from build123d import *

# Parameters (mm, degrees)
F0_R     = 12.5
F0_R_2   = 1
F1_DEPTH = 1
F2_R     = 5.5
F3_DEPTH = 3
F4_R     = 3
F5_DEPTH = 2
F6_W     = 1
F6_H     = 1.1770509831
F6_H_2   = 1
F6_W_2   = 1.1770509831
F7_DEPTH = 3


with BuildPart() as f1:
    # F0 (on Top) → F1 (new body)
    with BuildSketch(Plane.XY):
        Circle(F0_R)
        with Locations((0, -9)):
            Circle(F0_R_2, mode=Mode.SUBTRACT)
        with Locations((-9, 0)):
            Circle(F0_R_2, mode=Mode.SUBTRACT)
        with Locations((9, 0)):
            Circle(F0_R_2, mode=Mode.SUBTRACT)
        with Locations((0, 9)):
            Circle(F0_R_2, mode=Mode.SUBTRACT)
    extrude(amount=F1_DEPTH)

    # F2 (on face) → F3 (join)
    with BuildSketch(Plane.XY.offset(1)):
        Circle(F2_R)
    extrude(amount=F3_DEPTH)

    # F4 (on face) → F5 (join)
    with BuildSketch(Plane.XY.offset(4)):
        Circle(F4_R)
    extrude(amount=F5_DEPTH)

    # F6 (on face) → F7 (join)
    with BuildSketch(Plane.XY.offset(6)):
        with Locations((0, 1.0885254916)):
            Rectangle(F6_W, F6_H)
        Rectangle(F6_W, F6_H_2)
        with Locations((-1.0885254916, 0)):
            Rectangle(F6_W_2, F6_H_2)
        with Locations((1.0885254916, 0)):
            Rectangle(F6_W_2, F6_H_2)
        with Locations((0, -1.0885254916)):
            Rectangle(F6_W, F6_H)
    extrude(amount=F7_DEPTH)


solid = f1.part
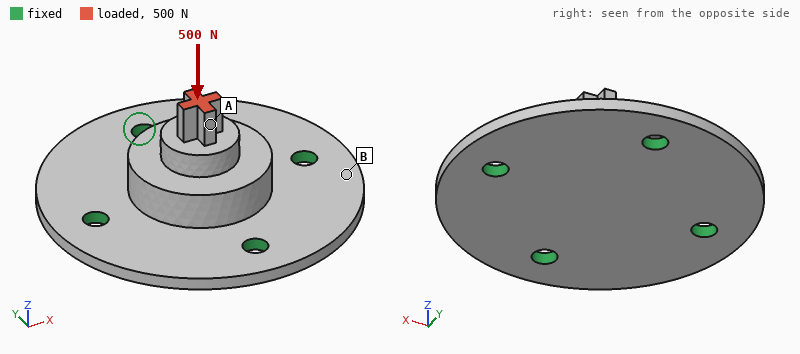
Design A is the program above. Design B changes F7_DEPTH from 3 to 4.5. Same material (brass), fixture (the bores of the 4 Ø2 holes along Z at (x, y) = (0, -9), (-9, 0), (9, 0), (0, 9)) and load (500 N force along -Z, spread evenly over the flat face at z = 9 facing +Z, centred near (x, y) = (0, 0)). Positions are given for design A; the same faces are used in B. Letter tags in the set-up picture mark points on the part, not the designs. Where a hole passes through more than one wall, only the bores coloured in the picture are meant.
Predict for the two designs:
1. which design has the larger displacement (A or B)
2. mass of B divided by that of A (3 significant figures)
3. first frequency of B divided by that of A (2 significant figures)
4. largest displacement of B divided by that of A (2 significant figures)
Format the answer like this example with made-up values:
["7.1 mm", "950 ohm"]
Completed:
["B", "1.01", "1.00", "1.1"]
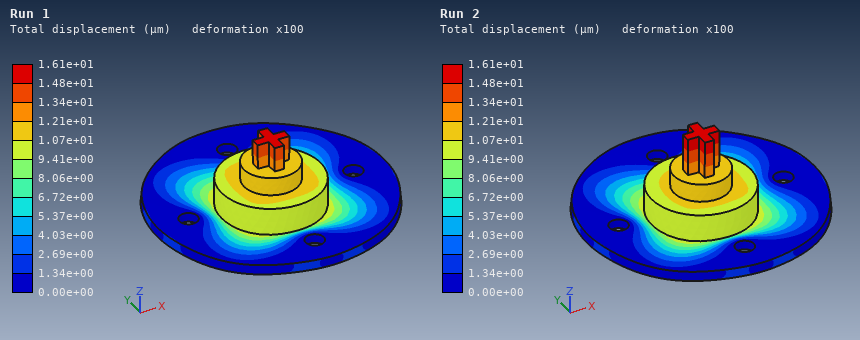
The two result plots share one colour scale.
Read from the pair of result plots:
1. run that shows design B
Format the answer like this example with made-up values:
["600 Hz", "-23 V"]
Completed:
["Run 2"]
